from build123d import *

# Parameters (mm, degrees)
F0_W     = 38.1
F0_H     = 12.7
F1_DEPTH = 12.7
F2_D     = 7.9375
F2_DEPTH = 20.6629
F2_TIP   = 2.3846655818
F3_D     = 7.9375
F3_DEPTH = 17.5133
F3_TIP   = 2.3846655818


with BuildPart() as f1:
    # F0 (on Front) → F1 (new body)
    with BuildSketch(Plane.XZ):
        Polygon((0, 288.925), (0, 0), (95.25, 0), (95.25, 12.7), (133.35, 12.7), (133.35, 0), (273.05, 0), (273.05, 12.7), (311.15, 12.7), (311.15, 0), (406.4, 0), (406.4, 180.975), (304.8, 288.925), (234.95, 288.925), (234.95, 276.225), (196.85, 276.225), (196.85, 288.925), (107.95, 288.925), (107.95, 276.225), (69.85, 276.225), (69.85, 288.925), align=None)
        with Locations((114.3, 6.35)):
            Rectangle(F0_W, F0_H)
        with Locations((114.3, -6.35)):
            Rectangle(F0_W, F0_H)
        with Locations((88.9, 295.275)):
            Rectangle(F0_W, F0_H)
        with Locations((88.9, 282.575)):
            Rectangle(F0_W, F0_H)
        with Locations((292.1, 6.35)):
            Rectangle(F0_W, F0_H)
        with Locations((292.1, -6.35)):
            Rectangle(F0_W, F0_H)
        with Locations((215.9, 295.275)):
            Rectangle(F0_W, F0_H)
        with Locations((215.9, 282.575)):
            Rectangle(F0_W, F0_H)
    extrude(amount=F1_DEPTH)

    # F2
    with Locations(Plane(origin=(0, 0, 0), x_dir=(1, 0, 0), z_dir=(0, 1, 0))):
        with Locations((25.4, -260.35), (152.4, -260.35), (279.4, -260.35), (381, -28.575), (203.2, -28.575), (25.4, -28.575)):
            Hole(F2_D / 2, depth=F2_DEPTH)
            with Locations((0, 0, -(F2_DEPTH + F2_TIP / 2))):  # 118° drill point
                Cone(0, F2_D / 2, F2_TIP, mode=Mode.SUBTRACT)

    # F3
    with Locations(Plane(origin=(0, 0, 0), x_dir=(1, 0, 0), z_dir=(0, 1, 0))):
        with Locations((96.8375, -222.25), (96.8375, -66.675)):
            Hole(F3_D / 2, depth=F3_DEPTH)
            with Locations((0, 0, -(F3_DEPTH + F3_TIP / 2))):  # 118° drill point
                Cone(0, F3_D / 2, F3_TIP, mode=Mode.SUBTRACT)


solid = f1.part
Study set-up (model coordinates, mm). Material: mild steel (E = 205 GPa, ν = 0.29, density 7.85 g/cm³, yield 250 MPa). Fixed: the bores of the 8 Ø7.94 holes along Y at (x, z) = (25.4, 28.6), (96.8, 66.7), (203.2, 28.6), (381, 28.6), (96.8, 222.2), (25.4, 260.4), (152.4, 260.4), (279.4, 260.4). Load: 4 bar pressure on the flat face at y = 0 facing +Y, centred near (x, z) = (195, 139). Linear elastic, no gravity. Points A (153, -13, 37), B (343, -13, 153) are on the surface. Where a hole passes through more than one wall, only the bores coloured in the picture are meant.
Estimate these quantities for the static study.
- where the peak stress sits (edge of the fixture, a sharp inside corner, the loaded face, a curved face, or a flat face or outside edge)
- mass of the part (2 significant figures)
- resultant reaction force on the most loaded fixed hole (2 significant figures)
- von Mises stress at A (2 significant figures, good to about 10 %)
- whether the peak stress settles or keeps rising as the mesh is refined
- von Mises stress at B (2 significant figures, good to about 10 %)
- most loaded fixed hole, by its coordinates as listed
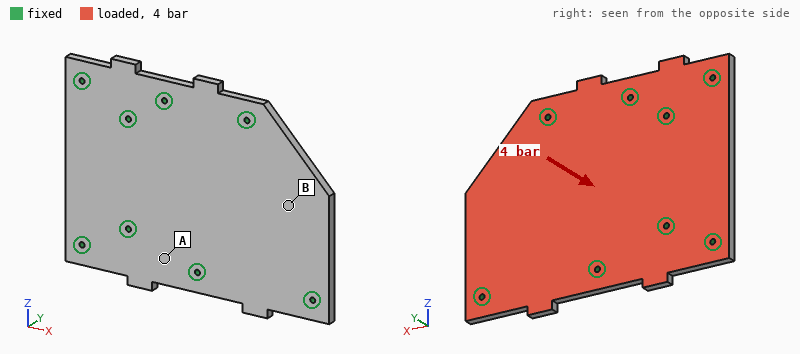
edge of the fixture
11 kg
9.2 kN
20 MPa
keeps rising
47 MPa
(279.4, 260.4)
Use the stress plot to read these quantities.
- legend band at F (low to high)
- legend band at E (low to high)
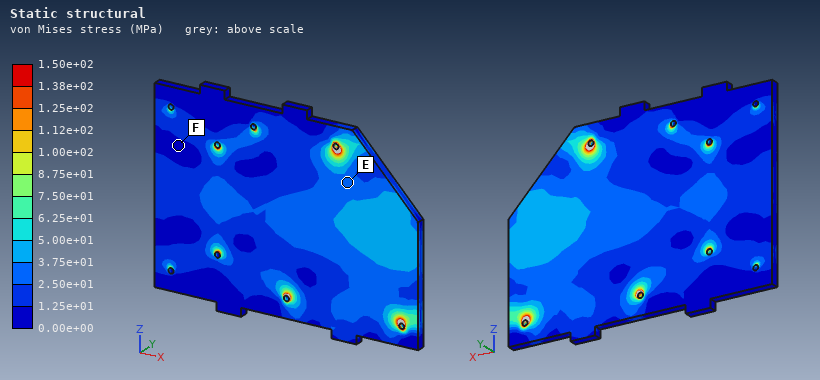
0.00e+00 to 1.25e+01 MPa
2.50e+01 to 3.75e+01 MPa
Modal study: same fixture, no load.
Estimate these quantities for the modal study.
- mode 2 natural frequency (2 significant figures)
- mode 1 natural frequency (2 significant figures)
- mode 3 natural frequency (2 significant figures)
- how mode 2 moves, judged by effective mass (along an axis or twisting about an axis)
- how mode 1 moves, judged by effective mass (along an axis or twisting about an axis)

1200 Hz
800 Hz
1500 Hz
along Y
along Y
